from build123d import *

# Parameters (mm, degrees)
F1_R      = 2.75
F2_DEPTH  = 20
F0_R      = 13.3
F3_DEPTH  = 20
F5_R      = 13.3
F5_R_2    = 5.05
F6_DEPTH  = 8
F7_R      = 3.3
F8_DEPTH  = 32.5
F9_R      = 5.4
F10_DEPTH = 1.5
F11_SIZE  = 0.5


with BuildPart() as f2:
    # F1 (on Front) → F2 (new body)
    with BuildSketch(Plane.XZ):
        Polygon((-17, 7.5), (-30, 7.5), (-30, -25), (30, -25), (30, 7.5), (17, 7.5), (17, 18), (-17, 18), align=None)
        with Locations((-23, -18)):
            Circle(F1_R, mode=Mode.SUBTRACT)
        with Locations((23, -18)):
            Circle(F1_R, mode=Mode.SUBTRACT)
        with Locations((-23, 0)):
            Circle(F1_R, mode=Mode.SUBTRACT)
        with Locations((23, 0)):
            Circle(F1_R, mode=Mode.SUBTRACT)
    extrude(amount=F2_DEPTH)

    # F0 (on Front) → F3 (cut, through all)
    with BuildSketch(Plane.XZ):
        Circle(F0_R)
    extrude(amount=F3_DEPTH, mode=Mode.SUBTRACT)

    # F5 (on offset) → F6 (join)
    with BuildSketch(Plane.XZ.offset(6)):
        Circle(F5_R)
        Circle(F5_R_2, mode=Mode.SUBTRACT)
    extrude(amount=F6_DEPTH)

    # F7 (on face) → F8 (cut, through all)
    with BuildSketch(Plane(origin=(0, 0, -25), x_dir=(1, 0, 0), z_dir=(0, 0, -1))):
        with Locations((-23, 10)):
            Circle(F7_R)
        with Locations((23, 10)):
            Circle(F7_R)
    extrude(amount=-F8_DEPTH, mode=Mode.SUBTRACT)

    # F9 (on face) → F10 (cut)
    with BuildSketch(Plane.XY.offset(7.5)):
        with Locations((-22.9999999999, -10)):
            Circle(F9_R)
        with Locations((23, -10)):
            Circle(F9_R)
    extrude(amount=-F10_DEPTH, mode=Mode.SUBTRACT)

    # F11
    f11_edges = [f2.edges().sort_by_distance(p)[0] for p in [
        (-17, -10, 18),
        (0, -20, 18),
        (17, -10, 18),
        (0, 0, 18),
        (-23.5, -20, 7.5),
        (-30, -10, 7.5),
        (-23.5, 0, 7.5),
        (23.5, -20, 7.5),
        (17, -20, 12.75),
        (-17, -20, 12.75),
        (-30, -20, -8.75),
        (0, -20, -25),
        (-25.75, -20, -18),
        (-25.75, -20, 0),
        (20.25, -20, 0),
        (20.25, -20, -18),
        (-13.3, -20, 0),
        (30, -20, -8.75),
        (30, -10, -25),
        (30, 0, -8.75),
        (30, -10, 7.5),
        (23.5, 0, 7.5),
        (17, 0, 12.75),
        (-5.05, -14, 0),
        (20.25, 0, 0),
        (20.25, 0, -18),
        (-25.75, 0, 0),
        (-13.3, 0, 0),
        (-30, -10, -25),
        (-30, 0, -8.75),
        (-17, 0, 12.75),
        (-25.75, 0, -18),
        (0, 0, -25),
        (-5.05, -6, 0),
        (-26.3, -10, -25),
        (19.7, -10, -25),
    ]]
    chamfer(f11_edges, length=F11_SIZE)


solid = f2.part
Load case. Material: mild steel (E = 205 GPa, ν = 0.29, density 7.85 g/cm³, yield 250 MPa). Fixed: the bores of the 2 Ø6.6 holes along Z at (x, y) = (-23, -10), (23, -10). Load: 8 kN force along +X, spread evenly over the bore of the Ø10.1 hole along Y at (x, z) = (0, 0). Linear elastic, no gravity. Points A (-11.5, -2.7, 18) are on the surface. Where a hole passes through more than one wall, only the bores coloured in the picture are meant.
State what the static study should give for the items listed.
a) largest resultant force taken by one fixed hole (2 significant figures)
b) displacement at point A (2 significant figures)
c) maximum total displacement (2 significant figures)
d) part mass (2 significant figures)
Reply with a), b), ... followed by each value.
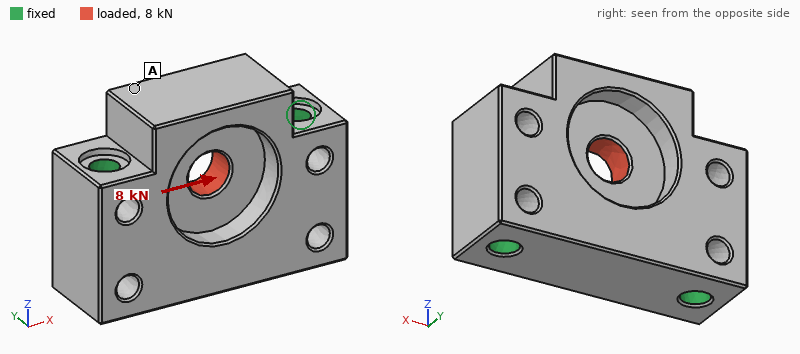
a) 4.1 kN
b) 1.3 µm
c) 2.6 µm
d) 270 g
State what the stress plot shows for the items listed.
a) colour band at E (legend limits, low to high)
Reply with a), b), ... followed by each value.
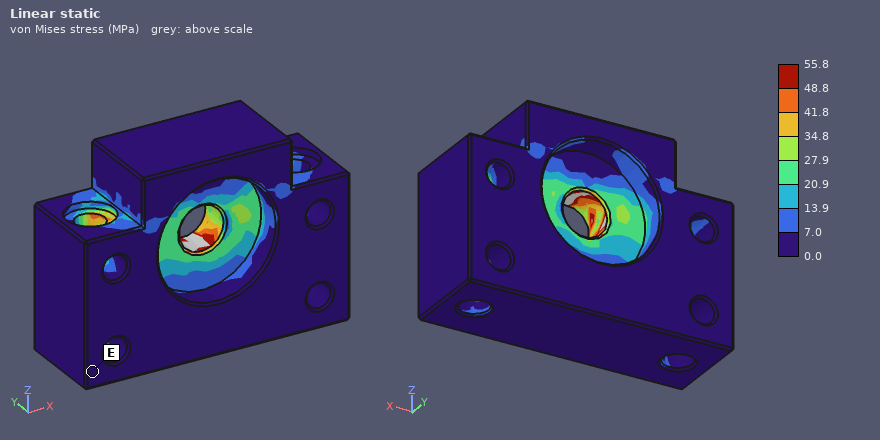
a) 0.0 to 7.0 MPa
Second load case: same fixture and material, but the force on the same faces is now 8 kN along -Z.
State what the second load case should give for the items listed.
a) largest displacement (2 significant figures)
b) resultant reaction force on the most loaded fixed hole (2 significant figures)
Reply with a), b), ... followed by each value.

a) 3.5 µm
b) 4.1 kN
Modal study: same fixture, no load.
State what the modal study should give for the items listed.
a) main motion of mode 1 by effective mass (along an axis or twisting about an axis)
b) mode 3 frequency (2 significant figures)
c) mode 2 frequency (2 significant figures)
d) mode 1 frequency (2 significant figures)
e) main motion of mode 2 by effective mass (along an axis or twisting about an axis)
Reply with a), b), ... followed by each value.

a) along Y
b) 27 kHz
c) 25 kHz
d) 15 kHz
e) along Y
